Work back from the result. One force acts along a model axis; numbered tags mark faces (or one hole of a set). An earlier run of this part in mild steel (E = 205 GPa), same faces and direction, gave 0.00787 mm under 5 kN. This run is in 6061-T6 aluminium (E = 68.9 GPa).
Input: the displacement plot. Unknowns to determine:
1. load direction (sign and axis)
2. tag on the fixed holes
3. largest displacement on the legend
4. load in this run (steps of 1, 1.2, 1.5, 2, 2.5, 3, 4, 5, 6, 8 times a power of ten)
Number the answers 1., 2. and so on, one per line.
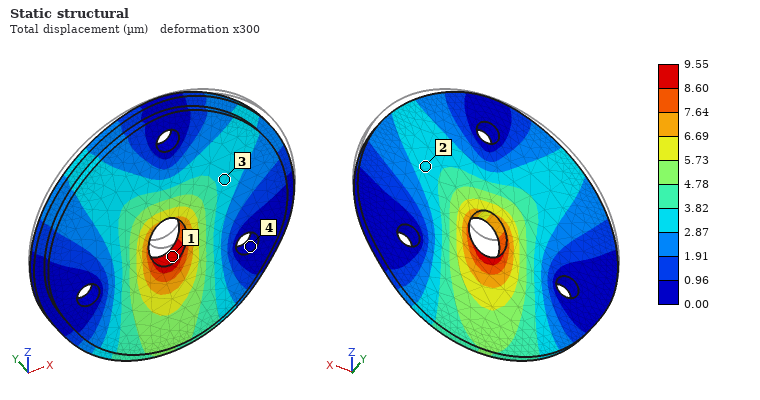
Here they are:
1. -Z
2. 4
3. 9.55 µm
4. 2 kN
